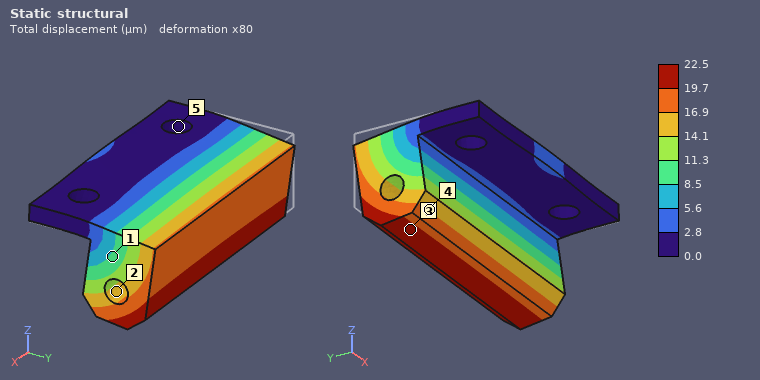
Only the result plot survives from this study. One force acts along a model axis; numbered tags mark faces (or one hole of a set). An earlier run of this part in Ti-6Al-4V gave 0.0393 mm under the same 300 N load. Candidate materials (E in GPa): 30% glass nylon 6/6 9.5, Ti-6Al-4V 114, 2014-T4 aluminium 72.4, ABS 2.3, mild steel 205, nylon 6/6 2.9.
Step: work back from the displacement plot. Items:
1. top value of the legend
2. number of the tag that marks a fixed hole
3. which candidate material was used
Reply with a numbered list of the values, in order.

1. 22.5 µm
2. 5
3. mild steel
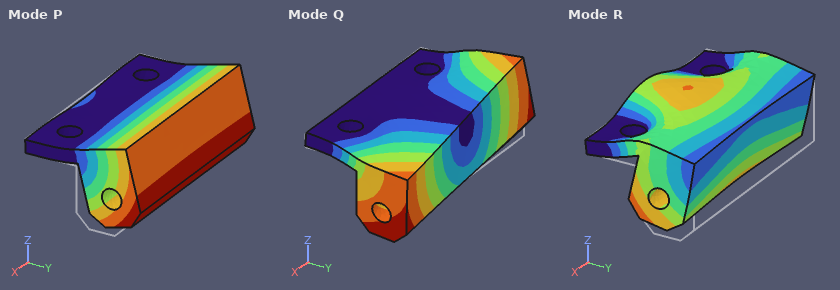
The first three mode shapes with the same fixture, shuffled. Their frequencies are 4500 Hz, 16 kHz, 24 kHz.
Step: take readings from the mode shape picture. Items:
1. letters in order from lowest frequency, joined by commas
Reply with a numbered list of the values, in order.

1. P, Q, R
